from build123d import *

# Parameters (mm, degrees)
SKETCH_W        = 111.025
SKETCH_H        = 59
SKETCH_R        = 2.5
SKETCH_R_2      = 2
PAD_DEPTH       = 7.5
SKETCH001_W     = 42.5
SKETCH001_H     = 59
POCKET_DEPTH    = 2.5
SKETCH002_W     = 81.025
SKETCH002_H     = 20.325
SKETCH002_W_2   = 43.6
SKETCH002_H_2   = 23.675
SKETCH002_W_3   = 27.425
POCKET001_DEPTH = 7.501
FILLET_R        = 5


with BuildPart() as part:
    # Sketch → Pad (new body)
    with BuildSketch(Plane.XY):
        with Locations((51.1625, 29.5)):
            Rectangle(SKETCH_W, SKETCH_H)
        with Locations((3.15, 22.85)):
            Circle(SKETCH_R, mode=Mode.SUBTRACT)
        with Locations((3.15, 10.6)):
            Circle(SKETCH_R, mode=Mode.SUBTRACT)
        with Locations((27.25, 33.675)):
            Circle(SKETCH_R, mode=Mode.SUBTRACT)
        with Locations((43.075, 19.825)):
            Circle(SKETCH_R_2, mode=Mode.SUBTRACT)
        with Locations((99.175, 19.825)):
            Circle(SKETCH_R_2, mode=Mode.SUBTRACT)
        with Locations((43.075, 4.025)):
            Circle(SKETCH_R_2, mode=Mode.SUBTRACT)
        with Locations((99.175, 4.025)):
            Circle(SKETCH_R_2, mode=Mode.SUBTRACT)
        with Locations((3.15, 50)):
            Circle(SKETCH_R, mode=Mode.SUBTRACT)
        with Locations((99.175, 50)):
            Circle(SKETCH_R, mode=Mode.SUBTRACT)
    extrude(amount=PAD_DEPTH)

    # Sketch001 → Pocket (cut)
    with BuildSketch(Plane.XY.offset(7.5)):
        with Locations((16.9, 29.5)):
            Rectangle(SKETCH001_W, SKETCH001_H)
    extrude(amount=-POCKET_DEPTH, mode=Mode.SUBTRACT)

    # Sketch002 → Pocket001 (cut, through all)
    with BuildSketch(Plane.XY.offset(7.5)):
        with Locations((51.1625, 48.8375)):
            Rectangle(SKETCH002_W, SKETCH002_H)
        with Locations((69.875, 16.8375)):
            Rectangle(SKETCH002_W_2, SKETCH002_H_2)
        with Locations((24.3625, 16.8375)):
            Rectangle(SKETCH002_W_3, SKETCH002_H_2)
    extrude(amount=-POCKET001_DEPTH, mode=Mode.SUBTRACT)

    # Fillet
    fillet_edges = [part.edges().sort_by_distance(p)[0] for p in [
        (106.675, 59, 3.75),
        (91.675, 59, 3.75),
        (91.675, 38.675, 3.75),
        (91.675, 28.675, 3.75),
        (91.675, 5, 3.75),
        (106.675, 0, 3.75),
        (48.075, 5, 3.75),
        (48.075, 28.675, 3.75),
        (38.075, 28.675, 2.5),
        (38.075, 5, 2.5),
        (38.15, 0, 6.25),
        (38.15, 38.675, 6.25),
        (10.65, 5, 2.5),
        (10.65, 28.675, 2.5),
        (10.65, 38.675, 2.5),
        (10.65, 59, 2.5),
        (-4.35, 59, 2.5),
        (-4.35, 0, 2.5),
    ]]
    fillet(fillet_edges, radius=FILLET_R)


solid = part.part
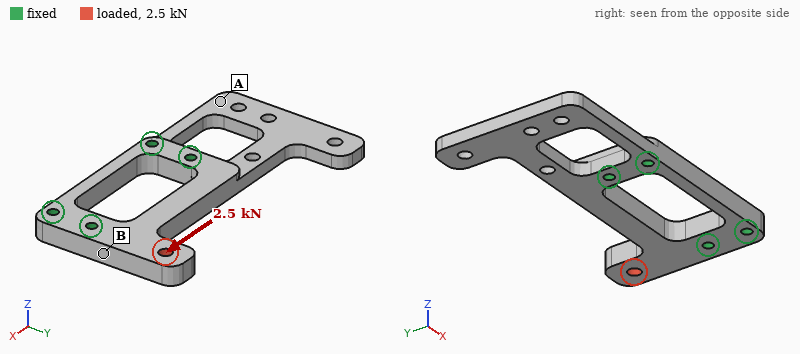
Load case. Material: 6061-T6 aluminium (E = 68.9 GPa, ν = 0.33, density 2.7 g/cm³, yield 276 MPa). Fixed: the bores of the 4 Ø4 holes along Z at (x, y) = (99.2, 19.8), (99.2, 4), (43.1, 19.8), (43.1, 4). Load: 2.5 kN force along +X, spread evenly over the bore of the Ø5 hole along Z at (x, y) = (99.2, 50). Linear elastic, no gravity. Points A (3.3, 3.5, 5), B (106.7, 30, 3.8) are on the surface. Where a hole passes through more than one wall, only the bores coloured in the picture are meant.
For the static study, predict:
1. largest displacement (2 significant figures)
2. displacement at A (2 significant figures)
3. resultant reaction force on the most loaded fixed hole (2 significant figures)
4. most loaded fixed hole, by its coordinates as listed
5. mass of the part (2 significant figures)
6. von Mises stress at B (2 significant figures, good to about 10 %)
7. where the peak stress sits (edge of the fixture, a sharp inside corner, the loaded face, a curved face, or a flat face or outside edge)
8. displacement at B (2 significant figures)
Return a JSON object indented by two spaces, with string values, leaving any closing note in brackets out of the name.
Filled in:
{
  "largest displacement": "0.16 mm",
  "displacement at A": "0.030 mm",
  "resultant reaction force on the most loaded fixed hole": "2.1 kN",
  "most loaded fixed hole, by its coordinates as listed": "(43.1, 19.8)",
  "mass of the part": "54 g",
  "von Mises stress at B": "81 MPa",
  "where the peak stress sits": "a curved face",
  "displacement at B": "0.032 mm"
}
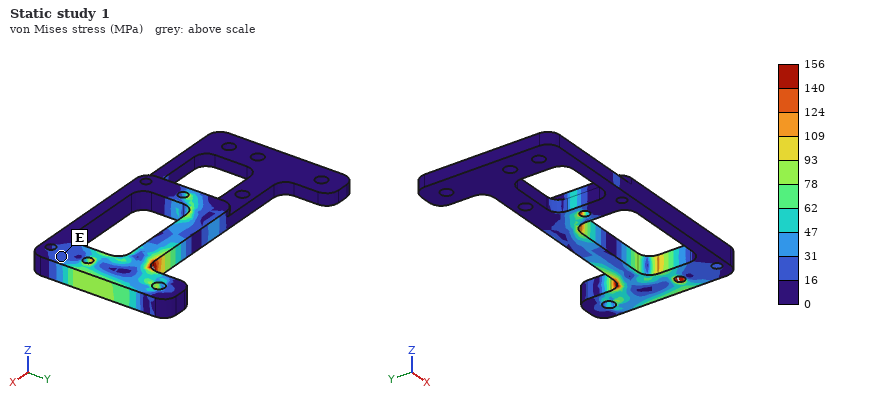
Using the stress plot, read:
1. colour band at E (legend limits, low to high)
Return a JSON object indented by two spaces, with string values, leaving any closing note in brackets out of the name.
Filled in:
{
  "colour band at E": "16 to 31 MPa"
}
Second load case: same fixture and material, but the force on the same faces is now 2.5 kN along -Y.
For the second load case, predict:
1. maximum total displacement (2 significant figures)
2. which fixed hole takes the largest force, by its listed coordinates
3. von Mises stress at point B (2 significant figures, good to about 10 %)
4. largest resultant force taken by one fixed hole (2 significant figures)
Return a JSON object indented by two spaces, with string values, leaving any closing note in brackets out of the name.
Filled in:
{
  "maximum total displacement": "13 µm",
  "which fixed hole takes the largest force, by its listed coordinates": "(99.2, 19.8)",
  "von Mises stress at point B": "24 MPa",
  "largest resultant force taken by one fixed hole": "2.2 kN"
}
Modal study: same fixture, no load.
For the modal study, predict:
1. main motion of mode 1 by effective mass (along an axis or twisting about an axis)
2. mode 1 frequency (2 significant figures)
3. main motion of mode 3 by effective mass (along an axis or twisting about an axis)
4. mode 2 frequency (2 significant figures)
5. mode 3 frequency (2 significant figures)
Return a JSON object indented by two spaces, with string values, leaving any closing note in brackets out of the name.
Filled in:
{
  "main motion of mode 1 by effective mass": "along Z",
  "mode 1 frequency": "1000 Hz",
  "main motion of mode 3 by effective mass": "along Y",
  "mode 2 frequency": "2200 Hz",
  "mode 3 frequency": "3300 Hz"
}
